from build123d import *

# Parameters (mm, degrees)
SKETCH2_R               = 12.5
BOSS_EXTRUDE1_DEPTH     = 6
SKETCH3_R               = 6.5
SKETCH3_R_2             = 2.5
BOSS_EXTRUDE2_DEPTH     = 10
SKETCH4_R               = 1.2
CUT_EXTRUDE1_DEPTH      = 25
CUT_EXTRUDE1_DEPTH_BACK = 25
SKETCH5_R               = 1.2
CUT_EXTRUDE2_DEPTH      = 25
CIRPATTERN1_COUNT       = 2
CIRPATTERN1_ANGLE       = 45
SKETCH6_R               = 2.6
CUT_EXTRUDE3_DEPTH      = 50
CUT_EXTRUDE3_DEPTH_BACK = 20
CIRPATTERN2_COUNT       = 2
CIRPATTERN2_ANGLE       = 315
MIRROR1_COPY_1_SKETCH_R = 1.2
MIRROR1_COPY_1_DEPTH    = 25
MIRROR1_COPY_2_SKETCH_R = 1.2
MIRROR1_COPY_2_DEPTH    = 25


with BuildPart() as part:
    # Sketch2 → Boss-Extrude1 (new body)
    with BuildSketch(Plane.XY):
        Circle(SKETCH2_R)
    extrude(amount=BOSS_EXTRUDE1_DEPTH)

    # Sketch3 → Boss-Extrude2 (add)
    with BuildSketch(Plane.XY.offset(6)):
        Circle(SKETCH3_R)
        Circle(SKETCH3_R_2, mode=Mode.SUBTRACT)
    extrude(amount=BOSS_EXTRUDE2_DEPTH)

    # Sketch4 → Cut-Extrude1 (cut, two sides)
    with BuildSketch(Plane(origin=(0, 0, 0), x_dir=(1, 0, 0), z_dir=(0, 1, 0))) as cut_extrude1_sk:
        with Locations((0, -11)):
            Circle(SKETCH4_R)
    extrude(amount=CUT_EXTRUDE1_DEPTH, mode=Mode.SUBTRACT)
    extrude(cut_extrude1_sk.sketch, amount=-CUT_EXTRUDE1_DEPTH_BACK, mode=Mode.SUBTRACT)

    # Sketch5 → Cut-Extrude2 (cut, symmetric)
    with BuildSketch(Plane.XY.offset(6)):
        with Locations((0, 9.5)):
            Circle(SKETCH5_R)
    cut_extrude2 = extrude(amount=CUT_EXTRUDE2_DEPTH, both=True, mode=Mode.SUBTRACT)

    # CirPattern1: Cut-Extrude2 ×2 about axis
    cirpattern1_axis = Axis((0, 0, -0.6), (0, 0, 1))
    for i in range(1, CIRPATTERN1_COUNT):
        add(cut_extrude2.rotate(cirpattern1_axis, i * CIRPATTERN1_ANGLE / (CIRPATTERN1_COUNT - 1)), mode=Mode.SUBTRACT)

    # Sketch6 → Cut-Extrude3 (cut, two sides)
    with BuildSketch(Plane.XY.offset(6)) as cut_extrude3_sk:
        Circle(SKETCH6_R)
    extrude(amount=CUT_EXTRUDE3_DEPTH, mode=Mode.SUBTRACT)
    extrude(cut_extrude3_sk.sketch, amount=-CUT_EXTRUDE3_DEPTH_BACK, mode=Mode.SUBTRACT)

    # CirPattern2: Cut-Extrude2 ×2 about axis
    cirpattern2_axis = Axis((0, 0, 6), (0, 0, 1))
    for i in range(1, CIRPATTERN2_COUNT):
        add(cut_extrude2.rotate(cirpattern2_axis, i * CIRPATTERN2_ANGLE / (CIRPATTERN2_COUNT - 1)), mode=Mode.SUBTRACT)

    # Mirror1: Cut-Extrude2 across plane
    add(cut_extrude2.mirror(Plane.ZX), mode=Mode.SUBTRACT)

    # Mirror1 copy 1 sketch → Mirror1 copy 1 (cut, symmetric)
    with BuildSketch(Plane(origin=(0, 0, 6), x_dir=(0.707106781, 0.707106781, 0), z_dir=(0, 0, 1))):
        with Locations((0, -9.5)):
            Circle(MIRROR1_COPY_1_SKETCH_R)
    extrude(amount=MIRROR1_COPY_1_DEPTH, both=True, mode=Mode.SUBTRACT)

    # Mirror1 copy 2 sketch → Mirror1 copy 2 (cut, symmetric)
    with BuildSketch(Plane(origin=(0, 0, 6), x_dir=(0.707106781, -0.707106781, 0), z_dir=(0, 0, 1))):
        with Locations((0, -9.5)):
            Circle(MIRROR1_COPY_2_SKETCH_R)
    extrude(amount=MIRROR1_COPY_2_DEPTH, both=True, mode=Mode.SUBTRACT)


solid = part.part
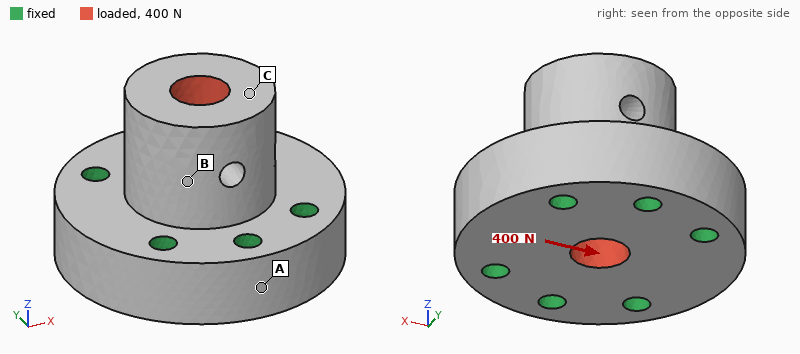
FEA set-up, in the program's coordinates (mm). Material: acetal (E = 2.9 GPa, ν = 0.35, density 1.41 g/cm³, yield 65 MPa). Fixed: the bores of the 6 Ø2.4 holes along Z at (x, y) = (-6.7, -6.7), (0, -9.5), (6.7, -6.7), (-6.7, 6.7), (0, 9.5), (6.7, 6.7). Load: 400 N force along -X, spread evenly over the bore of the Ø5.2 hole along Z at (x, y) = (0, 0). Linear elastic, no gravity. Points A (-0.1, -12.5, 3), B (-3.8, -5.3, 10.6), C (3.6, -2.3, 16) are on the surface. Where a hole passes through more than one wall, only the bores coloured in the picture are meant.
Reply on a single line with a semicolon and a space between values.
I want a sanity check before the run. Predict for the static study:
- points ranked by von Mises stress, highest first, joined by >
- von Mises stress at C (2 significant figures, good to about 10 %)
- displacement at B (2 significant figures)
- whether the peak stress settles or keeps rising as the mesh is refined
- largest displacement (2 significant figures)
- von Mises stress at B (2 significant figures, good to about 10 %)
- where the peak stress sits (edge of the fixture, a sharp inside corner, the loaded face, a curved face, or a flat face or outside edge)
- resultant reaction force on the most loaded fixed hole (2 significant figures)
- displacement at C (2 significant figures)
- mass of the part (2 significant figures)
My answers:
B > C > A; 2.3 MPa; 27 µm; keeps rising; 50 µm; 3.5 MPa; edge of the fixture; 120 N; 48 µm; 5.3 g
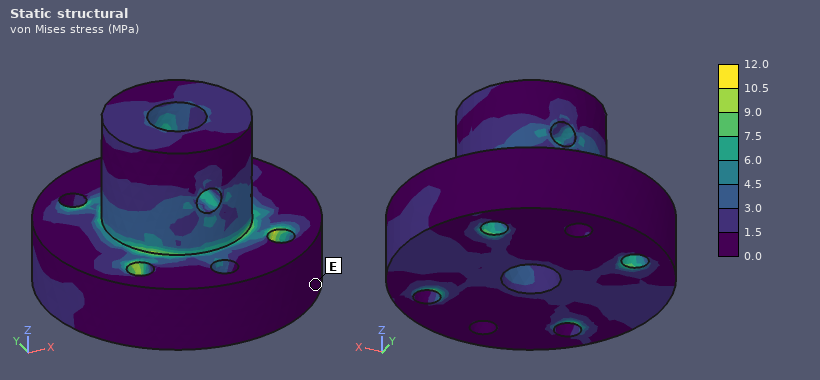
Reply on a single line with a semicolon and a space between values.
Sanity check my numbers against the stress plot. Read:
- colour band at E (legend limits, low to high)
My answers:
0.0 to 1.5 MPa
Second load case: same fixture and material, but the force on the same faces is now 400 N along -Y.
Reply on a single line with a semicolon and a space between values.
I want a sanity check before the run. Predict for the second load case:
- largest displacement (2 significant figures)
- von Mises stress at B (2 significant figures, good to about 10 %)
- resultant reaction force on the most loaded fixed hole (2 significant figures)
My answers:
41 µm; 1.6 MPa; 100 N
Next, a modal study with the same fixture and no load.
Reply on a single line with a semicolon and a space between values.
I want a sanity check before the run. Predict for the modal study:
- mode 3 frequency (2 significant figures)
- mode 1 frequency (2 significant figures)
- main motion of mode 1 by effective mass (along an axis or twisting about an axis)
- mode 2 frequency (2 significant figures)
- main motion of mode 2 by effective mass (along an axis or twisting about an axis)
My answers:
18 kHz; 11 kHz; along X; 12 kHz; along Y
